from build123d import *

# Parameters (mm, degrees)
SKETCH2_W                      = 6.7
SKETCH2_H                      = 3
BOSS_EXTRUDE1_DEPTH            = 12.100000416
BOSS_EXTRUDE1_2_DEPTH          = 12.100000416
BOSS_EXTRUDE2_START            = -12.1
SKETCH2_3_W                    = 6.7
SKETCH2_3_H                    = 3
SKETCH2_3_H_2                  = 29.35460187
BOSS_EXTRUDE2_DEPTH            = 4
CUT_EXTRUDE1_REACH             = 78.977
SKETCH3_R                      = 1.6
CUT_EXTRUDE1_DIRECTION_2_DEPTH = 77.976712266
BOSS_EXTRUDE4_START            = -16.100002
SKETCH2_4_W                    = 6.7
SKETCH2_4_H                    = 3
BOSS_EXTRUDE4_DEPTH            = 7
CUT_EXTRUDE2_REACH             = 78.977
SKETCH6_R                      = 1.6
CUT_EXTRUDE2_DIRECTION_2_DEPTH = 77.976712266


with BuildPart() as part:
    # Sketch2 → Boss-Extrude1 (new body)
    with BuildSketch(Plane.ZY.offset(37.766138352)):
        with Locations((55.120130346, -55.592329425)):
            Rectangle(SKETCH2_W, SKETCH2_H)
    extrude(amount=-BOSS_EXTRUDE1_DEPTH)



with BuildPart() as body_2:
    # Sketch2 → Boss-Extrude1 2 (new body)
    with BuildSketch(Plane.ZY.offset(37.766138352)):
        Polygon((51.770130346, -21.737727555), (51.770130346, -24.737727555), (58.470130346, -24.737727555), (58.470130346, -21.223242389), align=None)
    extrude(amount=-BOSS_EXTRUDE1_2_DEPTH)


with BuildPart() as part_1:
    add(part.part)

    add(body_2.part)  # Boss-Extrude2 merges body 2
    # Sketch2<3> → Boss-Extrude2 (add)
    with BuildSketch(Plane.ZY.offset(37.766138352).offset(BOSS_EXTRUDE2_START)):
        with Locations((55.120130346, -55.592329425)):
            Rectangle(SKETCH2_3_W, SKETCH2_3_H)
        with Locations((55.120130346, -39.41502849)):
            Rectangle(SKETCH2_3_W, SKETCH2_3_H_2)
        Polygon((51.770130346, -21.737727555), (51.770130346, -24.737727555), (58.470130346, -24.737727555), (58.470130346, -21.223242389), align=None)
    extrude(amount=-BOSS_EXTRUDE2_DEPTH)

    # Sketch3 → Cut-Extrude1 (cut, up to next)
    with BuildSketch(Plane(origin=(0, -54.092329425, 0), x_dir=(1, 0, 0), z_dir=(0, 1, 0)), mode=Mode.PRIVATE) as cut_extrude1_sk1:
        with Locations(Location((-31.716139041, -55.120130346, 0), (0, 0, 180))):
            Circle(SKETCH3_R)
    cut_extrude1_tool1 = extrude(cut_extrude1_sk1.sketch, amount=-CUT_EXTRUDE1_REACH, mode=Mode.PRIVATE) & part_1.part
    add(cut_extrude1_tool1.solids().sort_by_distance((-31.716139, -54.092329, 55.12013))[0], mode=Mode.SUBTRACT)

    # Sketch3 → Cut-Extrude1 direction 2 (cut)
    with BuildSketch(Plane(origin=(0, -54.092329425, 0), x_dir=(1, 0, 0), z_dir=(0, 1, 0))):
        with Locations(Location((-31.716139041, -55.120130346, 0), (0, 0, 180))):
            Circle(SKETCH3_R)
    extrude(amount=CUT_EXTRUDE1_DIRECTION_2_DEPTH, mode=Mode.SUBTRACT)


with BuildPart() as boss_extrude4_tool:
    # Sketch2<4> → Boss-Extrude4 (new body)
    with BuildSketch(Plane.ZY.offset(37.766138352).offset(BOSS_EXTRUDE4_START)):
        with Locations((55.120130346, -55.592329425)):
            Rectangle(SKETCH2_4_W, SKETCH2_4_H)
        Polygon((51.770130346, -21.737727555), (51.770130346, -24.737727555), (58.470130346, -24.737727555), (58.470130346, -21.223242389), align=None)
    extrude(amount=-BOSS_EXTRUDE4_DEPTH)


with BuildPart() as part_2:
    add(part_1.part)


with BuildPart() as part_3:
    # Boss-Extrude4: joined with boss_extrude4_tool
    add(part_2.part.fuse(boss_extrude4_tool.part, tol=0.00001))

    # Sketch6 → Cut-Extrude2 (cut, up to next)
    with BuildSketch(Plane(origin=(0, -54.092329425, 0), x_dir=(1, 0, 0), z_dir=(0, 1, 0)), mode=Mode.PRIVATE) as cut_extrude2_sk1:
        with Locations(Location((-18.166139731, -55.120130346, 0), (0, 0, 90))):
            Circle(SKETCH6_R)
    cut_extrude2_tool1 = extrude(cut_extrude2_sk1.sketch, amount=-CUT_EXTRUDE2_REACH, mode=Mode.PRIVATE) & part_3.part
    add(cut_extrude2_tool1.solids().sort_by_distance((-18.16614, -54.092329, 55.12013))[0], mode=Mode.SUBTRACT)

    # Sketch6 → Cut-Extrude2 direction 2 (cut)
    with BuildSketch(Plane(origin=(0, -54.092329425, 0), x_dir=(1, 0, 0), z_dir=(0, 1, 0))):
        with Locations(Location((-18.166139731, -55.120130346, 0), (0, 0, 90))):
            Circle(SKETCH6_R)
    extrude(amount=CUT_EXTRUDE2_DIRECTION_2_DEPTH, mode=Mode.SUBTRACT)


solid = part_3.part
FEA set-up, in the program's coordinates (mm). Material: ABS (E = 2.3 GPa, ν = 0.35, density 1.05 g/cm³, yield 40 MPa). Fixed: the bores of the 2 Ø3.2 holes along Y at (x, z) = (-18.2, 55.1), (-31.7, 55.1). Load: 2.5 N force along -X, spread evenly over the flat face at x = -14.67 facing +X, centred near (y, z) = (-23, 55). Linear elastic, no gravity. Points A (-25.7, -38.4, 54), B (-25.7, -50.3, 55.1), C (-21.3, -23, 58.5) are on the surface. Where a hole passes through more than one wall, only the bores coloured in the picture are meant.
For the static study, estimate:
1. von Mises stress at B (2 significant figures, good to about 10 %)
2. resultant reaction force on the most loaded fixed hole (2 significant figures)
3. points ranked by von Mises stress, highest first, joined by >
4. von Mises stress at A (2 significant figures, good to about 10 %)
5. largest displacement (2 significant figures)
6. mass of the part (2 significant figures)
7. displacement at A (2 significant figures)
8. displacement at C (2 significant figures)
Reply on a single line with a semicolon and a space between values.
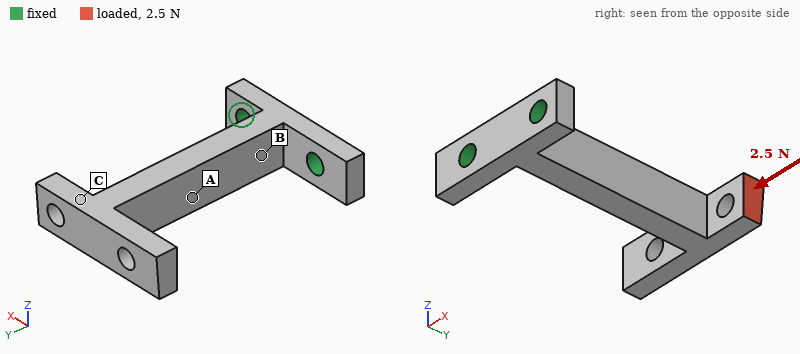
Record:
3.8 MPa; 9.0 N; B > A > C; 2.1 MPa; 0.46 mm; 1.7 g; 0.13 mm; 0.37 mm
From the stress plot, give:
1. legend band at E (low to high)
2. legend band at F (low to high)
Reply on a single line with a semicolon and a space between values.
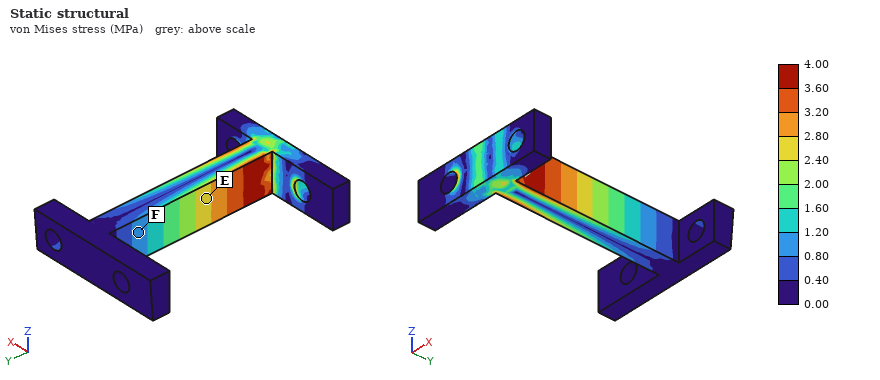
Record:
2.40 to 2.80 MPa; 0.80 to 1.20 MPa
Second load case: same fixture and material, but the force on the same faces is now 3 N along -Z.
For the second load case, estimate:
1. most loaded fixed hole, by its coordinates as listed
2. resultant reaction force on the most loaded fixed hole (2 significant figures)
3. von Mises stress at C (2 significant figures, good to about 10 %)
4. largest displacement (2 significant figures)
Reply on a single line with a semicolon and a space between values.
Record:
(-18.2, 55.1); 4.5 N; 0.88 MPa; 0.40 mm
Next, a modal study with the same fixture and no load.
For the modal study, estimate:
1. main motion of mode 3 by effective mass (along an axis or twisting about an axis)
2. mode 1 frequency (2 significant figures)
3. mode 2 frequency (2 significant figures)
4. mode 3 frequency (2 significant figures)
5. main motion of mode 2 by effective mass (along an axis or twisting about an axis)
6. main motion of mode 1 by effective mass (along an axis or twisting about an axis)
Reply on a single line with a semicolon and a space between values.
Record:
twisting about Y; 490 Hz; 620 Hz; 1600 Hz; along Z; along X
